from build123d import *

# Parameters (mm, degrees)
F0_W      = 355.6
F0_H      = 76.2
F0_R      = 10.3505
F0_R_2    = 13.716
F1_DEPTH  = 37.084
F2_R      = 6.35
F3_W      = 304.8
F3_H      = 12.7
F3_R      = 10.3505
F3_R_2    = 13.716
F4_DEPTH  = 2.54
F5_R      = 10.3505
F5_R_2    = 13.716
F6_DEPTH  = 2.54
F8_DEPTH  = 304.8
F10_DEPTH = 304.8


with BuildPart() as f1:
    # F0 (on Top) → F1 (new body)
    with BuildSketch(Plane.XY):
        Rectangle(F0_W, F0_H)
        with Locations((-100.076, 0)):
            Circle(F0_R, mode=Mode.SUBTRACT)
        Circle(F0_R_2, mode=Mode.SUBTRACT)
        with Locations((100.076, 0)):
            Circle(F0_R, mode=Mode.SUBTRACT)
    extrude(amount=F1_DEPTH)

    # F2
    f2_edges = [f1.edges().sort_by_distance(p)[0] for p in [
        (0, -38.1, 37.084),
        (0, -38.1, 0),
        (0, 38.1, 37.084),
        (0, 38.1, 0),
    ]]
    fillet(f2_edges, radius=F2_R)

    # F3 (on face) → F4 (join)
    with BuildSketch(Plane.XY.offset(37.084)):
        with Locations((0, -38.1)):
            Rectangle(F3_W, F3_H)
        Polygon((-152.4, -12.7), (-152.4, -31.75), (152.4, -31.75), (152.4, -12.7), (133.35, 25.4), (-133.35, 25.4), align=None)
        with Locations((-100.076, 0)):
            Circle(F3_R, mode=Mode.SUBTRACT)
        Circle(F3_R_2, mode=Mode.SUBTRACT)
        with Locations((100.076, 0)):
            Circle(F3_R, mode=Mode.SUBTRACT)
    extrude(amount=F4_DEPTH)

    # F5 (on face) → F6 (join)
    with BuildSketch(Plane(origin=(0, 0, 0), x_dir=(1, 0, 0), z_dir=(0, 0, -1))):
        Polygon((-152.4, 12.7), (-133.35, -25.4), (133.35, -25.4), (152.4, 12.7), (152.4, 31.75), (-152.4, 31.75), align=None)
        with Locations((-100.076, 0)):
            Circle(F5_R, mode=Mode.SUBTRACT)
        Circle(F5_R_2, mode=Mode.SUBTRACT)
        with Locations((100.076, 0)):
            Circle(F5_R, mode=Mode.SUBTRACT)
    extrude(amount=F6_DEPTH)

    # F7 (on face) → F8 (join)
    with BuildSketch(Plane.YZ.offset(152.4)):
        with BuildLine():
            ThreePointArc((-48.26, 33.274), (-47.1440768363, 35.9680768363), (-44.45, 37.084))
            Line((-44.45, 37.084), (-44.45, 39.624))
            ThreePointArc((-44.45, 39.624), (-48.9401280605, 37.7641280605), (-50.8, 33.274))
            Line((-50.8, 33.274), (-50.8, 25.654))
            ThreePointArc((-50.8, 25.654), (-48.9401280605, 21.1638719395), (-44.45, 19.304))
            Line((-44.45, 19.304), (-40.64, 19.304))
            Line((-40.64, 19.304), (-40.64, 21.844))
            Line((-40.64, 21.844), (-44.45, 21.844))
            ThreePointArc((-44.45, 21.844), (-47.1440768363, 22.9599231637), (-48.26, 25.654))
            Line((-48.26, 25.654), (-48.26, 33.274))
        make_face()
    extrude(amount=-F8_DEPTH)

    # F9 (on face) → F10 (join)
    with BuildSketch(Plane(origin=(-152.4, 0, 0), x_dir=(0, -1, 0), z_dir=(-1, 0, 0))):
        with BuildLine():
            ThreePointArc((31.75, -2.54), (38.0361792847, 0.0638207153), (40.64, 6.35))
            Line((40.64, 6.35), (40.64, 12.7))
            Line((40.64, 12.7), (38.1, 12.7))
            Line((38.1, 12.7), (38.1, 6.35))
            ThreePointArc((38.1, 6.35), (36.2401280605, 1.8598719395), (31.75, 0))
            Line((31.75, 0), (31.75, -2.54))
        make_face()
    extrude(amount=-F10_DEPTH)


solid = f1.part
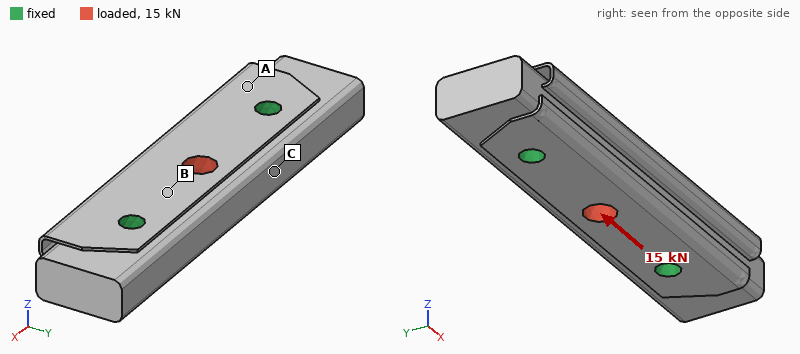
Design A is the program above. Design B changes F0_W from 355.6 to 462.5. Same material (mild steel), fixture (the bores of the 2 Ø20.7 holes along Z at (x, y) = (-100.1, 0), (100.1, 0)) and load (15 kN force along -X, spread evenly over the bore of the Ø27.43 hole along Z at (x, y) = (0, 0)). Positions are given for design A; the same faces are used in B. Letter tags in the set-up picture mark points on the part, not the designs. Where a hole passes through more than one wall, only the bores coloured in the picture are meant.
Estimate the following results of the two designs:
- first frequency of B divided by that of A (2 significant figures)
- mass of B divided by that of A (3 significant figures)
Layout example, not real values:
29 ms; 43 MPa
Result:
1.0; 1.28
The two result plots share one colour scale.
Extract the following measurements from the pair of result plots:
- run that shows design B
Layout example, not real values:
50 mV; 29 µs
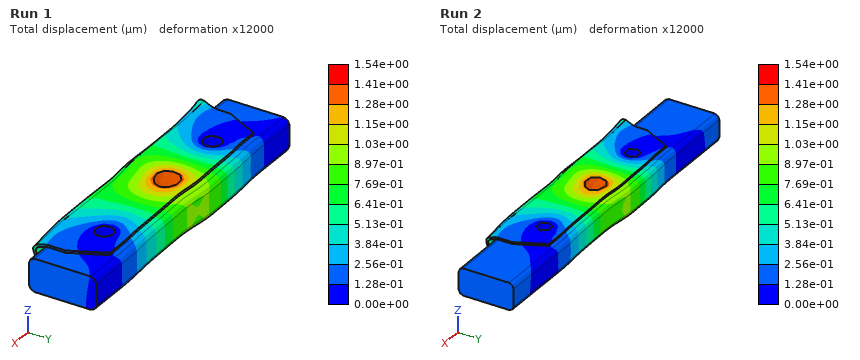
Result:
Run 2
